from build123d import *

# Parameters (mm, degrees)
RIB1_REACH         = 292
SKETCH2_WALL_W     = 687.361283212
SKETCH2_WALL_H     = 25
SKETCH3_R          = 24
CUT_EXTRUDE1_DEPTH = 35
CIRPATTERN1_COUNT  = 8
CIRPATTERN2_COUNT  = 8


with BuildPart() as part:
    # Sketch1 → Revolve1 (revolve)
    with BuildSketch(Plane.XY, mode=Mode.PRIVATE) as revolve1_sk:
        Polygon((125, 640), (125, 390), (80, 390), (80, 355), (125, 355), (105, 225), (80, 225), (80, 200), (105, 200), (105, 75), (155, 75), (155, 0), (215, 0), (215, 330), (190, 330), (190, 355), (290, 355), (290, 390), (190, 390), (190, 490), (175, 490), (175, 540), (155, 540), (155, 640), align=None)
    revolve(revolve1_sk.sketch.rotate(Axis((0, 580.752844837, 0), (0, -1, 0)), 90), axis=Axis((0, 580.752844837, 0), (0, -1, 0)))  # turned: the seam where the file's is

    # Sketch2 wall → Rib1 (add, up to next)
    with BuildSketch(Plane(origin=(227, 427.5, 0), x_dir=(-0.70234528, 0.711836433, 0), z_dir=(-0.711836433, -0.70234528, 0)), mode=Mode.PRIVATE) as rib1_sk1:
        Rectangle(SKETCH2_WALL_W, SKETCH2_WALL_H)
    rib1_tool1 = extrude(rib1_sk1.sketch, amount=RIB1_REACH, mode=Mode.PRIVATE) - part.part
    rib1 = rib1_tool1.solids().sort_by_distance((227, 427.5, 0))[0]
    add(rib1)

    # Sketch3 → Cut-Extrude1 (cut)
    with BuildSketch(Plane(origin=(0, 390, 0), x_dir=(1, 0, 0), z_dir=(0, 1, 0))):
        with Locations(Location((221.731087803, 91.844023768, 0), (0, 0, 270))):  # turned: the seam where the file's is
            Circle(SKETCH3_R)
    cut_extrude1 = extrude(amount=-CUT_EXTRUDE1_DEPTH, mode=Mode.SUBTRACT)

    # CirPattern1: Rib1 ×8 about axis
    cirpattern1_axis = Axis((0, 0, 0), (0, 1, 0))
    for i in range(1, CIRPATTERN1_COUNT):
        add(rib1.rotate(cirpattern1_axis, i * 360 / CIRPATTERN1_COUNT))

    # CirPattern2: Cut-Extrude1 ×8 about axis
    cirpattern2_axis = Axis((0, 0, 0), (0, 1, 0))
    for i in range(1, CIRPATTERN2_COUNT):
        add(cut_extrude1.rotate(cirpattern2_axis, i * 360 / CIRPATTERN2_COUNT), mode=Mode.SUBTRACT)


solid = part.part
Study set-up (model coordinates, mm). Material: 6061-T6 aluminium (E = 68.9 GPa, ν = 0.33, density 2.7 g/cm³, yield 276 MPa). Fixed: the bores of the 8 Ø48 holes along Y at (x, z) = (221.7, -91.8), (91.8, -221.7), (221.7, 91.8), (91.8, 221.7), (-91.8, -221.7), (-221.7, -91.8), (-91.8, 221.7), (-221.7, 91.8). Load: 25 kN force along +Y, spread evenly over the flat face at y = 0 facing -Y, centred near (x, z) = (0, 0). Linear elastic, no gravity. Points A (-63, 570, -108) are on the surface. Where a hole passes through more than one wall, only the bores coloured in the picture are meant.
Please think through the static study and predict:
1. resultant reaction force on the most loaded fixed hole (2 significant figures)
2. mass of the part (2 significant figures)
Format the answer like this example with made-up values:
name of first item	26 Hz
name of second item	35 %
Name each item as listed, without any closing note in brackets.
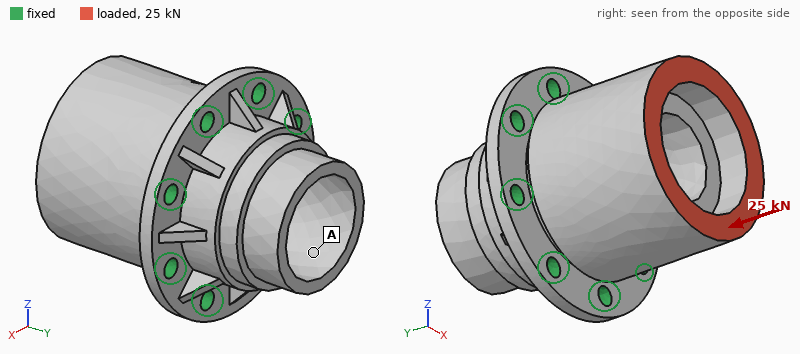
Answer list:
resultant reaction force on the most loaded fixed hole	3.1 kN
mass of the part	150 kg
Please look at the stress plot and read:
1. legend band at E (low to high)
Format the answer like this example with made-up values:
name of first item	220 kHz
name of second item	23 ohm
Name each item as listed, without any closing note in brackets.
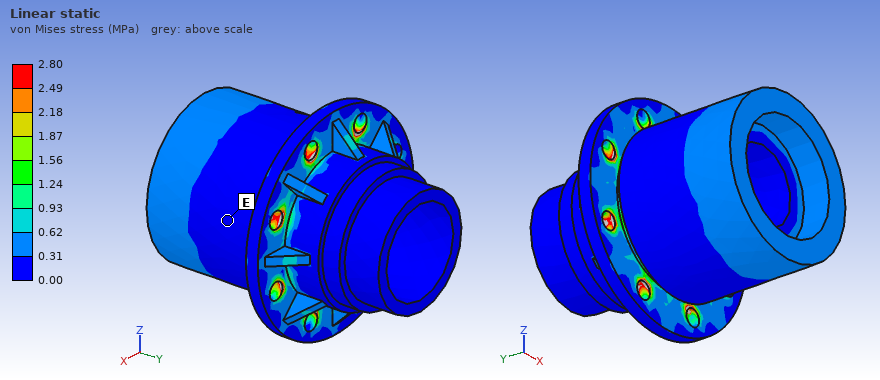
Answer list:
legend band at E	0.00 to 0.31 MPa
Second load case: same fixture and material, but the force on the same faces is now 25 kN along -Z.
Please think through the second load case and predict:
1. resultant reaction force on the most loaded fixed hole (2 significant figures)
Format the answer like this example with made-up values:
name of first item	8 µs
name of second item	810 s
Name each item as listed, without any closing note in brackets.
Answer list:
resultant reaction force on the most loaded fixed hole	11 kN
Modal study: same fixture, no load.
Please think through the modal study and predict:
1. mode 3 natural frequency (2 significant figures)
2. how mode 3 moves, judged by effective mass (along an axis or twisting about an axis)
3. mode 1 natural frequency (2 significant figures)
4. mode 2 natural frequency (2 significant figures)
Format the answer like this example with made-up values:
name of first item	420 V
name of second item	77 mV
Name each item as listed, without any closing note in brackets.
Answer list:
mode 3 natural frequency	1400 Hz
how mode 3 moves, judged by effective mass	along Y
mode 1 natural frequency	820 Hz
mode 2 natural frequency	820 Hz
